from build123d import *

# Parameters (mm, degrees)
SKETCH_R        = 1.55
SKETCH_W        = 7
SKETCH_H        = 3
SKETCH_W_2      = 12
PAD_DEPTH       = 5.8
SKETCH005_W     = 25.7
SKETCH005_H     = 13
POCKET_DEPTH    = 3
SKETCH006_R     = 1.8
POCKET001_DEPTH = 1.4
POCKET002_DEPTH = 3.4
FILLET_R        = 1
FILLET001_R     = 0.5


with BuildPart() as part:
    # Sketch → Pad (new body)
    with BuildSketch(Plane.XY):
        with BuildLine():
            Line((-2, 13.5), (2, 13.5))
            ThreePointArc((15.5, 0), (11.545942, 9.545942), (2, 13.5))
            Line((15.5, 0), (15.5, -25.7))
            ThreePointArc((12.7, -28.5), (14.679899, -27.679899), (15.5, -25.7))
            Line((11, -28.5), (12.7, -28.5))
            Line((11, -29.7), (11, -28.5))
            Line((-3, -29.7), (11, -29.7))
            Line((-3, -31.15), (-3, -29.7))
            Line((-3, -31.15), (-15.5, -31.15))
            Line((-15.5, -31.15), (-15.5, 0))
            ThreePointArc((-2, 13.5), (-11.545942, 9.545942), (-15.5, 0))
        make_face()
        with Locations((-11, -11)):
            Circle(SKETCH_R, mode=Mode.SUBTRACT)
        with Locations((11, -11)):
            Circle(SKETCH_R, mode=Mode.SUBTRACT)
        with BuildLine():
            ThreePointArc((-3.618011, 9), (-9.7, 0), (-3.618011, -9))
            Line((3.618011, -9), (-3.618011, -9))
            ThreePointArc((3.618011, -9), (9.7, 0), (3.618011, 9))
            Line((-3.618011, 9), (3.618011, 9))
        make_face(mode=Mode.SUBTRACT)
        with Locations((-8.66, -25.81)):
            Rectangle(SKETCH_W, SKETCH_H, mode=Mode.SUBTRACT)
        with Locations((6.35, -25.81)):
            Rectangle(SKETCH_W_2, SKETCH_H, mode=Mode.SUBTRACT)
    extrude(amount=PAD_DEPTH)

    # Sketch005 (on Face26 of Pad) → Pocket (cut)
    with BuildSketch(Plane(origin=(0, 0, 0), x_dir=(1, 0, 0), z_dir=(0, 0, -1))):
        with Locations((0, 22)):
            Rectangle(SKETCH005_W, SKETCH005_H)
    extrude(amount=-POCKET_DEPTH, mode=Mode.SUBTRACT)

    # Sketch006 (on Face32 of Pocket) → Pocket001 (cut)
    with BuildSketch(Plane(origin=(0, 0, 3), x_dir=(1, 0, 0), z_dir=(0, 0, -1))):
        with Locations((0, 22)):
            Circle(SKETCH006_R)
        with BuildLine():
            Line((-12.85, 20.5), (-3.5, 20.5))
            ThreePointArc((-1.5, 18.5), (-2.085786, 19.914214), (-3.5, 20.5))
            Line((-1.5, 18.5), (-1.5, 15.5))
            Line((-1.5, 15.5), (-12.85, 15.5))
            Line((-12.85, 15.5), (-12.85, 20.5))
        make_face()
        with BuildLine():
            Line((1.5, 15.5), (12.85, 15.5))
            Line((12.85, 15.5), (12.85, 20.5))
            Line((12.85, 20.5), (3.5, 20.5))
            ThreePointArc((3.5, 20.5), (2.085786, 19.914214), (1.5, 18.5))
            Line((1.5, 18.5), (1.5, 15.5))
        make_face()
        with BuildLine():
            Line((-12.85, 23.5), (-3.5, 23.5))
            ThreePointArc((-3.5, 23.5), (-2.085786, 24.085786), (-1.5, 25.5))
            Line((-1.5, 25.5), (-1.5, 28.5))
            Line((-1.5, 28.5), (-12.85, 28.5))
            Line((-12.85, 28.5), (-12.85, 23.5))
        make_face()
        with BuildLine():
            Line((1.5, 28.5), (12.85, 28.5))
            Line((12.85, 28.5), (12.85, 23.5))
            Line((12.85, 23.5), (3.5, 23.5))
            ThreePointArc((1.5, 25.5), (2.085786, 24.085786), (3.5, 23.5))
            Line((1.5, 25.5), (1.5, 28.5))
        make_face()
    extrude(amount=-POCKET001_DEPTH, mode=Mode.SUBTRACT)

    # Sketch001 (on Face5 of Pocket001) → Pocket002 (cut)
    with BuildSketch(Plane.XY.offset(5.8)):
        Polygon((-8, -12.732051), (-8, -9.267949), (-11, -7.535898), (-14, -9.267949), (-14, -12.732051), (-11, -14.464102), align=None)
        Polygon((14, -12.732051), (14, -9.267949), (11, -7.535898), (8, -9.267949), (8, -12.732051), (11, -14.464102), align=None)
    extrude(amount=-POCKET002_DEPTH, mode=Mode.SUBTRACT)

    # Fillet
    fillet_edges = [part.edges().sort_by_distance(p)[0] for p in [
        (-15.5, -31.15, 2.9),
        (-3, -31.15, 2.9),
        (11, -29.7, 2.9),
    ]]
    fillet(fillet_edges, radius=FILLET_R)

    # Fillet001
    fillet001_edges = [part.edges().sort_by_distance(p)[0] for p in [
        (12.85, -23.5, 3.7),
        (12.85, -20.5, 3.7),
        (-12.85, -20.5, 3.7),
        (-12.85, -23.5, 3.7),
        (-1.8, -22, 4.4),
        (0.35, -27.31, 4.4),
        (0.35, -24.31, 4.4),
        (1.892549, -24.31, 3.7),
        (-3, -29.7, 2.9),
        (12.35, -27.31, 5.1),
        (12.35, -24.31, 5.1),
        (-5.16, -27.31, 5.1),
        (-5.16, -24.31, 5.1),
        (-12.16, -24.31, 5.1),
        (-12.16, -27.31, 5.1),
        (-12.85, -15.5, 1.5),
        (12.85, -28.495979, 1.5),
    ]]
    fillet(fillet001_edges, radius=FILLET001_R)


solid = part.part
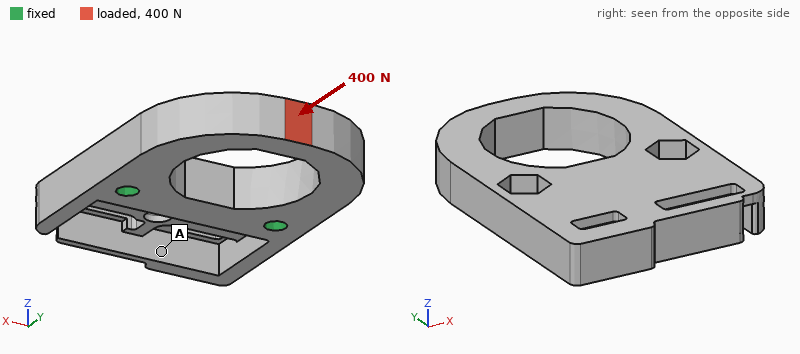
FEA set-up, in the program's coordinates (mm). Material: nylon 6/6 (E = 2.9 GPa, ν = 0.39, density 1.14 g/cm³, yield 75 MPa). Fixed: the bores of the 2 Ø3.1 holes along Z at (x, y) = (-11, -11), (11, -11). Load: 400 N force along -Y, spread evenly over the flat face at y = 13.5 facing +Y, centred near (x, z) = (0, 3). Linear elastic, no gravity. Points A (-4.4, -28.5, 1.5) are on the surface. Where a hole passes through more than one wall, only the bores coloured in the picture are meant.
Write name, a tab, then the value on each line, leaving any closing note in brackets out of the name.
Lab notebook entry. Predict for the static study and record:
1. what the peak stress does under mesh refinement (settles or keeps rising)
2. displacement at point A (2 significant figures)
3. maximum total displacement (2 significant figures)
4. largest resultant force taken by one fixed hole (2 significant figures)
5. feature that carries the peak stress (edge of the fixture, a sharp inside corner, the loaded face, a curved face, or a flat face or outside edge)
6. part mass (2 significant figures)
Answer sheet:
what the peak stress does under mesh refinement	keeps rising
displacement at point A	0.099 mm
maximum total displacement	0.45 mm
largest resultant force taken by one fixed hole	210 N
feature that carries the peak stress	edge of the fixture
part mass	4.6 g
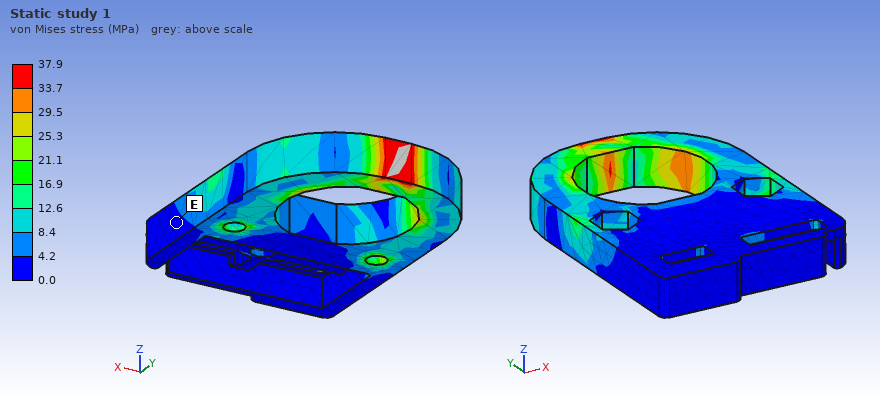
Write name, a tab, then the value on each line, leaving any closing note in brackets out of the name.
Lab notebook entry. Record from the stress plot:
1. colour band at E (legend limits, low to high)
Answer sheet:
colour band at E	0.0 to 4.2 MPa
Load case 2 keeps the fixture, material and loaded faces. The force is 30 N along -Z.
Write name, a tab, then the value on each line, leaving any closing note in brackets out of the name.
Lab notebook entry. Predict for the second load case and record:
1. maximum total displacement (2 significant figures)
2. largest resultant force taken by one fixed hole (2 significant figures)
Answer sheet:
maximum total displacement	0.50 mm
largest resultant force taken by one fixed hole	15 N
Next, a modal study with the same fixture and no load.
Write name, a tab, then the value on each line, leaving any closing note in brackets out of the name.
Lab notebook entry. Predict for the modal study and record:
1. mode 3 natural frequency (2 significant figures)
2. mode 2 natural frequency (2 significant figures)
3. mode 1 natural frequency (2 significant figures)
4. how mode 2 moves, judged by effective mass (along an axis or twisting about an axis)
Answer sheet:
mode 3 natural frequency	3100 Hz
mode 2 natural frequency	2300 Hz
mode 1 natural frequency	1500 Hz
how mode 2 moves, judged by effective mass	along Z
